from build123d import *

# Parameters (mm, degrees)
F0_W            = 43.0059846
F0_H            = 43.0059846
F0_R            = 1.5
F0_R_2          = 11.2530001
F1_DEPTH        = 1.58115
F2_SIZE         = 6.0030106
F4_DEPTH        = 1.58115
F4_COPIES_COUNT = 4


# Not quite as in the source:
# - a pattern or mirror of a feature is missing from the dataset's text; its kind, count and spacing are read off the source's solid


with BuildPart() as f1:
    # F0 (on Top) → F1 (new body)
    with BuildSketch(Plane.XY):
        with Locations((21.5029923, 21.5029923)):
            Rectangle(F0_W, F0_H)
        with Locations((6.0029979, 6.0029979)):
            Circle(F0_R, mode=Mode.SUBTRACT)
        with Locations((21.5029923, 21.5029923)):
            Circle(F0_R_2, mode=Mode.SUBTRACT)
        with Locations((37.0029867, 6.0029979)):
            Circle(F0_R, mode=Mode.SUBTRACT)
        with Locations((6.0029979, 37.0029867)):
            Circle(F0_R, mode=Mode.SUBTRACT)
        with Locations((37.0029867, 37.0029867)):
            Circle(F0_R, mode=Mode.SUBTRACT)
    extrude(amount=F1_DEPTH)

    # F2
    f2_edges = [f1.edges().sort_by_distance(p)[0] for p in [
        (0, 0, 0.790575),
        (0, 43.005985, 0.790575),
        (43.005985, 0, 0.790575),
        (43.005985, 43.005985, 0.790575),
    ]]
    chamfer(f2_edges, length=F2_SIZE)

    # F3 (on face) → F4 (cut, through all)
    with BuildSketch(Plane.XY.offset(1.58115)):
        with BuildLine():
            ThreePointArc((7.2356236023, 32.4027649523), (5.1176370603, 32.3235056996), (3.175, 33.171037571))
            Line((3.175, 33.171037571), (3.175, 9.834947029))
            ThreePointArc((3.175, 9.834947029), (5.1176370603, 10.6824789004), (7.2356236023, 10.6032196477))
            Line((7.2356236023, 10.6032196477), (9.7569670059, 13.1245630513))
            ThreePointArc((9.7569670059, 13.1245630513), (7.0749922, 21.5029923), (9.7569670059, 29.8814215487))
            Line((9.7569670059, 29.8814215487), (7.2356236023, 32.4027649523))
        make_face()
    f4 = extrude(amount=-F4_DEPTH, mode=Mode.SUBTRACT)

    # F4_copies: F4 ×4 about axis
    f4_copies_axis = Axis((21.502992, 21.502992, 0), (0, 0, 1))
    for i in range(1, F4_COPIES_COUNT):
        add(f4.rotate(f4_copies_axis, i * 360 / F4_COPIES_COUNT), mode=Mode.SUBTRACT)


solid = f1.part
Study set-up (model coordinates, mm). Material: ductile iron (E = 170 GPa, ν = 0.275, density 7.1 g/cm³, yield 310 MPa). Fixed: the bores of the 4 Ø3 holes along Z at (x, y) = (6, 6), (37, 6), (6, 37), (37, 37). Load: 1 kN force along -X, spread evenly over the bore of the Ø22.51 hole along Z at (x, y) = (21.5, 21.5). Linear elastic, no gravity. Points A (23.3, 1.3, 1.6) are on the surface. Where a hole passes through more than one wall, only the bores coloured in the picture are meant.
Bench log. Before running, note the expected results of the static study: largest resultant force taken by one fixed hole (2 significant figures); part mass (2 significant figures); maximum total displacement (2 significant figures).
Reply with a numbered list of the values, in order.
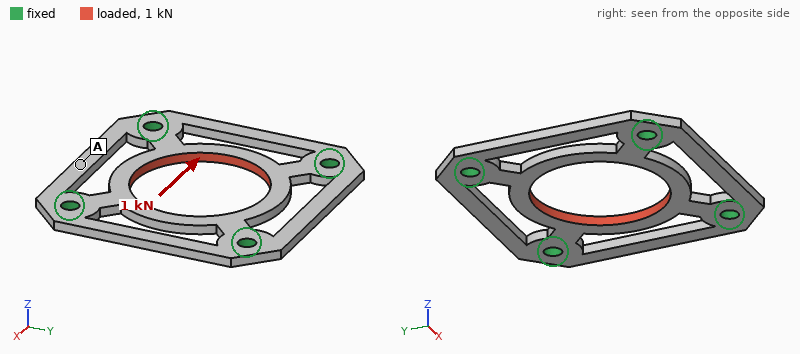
1. 250 N
2. 10 g
3. 17 µm
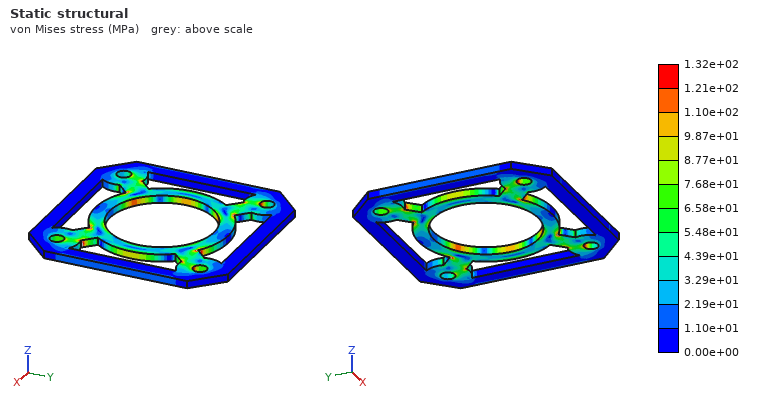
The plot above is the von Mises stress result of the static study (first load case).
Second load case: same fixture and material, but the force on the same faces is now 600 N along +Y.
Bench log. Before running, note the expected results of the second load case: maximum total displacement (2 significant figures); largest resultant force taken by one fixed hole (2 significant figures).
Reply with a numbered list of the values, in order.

1. 10 µm
2. 150 N
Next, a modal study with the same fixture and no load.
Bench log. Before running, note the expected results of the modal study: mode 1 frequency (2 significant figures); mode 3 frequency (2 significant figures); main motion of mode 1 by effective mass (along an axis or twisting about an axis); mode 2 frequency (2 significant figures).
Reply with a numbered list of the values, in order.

1. 8300 Hz
2. 9000 Hz
3. along Z
4. 9000 Hz
